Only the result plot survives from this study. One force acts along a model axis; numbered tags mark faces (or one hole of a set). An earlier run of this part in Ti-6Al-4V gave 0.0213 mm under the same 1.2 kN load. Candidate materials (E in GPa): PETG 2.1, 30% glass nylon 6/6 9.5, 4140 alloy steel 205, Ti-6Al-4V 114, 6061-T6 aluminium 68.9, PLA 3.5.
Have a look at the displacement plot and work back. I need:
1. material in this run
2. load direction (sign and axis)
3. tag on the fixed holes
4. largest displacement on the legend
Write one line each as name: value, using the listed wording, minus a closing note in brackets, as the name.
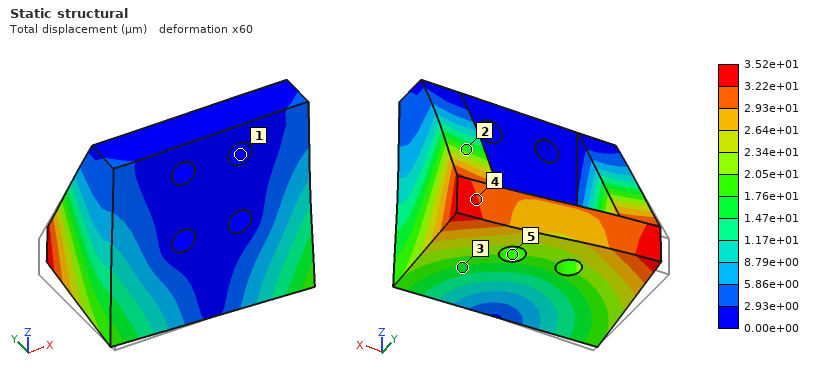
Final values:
material in this run: 6061-T6 aluminium
load direction: +X
tag on the fixed holes: 1
largest displacement on the legend: 3.52e+01 µm
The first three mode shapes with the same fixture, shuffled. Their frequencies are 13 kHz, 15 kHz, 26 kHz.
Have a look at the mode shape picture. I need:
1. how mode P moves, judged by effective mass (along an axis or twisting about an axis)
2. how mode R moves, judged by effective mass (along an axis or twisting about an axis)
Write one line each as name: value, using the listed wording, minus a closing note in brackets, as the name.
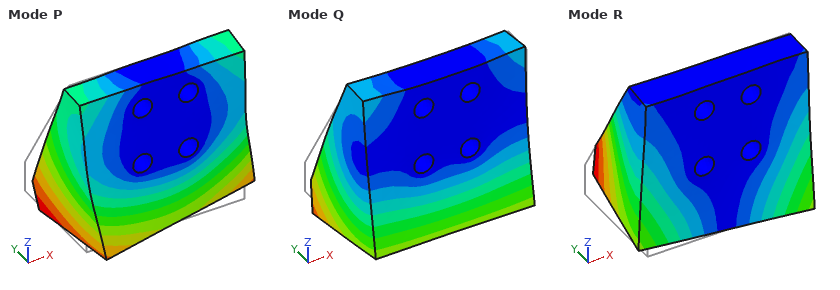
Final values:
how mode P moves, judged by effective mass: along X
how mode R moves, judged by effective mass: along X
